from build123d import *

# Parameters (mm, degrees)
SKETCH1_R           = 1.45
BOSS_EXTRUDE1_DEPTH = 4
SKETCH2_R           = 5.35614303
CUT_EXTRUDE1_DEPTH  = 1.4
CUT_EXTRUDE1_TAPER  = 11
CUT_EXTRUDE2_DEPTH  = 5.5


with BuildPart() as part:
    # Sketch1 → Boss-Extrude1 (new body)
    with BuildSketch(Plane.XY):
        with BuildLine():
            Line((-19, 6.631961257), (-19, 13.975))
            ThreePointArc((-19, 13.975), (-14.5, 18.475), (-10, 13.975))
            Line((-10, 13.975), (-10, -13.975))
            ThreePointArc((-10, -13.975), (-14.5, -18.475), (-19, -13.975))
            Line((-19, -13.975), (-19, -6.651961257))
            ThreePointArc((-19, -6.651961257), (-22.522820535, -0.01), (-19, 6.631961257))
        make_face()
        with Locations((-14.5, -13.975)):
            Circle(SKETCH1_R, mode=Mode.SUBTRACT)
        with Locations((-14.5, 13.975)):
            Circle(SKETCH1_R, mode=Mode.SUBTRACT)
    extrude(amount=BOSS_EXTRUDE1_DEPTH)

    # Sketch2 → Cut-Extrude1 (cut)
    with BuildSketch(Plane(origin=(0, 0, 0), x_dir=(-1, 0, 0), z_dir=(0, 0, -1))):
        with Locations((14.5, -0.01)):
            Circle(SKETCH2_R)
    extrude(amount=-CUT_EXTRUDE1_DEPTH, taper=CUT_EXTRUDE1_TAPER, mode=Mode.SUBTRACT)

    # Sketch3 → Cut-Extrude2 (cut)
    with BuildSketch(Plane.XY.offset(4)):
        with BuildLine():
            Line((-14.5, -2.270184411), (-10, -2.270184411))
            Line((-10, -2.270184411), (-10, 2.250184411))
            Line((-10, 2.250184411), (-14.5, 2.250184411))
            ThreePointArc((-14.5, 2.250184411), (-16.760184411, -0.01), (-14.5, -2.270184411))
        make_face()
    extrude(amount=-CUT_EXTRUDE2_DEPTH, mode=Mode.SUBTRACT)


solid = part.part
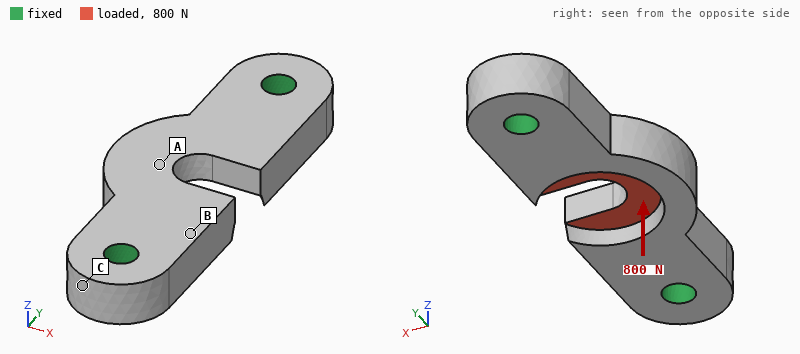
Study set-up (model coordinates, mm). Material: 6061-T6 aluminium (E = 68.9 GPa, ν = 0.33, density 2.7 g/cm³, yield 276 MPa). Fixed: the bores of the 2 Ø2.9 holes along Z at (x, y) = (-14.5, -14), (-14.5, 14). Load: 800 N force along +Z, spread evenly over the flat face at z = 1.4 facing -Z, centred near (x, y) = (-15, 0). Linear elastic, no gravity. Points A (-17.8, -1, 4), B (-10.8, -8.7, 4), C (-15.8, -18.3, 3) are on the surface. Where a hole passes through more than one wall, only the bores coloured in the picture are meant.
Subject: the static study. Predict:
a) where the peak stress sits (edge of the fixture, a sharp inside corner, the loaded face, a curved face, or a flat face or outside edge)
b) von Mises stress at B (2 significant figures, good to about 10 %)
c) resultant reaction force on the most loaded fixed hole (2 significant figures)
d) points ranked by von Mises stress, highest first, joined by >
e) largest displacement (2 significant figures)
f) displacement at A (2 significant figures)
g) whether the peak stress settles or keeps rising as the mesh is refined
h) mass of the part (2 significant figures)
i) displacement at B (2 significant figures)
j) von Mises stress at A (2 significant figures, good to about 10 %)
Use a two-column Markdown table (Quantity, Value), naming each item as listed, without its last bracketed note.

| Quantity | Value |
|---|---|
| where the peak stress sits | edge of the fixture |
| von Mises stress at B | 55 MPa |
| resultant reaction force on the most loaded fixed hole | 420 N |
| points ranked by von Mises stress, highest first, joined by > | A > B > C |
| largest displacement | 42 µm |
| displacement at A | 40 µm |
| whether the peak stress settles or keeps rising as the mesh is refined | keeps rising |
| mass of the part | 3.1 g |
| displacement at B | 12 µm |
| von Mises stress at A | 110 MPa |
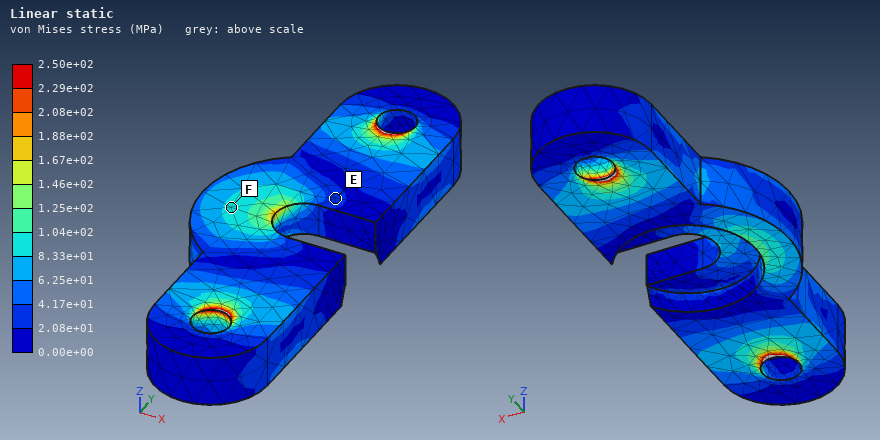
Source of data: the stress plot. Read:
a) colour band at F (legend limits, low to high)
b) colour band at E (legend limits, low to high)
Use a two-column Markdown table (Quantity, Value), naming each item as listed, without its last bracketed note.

| Quantity | Value |
|---|---|
| colour band at F | 8.33e+01 to 1.04e+02 MPa |
| colour band at E | 2.08e+01 to 4.17e+01 MPa |
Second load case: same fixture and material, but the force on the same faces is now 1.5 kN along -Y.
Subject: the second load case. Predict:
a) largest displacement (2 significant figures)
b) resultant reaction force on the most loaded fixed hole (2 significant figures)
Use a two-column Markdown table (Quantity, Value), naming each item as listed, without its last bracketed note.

| Quantity | Value |
|---|---|
| largest displacement | 6.8 µm |
| resultant reaction force on the most loaded fixed hole | 750 N |
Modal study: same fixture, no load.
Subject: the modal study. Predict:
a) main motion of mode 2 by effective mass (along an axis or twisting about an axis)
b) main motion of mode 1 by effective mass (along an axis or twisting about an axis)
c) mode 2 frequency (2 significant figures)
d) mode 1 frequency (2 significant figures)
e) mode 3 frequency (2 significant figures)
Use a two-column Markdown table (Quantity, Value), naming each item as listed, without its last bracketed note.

| Quantity | Value |
|---|---|
| main motion of mode 2 by effective mass | along X |
| main motion of mode 1 by effective mass | along Z |
| mode 2 frequency | 35 kHz |
| mode 1 frequency | 21 kHz |
| mode 3 frequency | 37 kHz |
